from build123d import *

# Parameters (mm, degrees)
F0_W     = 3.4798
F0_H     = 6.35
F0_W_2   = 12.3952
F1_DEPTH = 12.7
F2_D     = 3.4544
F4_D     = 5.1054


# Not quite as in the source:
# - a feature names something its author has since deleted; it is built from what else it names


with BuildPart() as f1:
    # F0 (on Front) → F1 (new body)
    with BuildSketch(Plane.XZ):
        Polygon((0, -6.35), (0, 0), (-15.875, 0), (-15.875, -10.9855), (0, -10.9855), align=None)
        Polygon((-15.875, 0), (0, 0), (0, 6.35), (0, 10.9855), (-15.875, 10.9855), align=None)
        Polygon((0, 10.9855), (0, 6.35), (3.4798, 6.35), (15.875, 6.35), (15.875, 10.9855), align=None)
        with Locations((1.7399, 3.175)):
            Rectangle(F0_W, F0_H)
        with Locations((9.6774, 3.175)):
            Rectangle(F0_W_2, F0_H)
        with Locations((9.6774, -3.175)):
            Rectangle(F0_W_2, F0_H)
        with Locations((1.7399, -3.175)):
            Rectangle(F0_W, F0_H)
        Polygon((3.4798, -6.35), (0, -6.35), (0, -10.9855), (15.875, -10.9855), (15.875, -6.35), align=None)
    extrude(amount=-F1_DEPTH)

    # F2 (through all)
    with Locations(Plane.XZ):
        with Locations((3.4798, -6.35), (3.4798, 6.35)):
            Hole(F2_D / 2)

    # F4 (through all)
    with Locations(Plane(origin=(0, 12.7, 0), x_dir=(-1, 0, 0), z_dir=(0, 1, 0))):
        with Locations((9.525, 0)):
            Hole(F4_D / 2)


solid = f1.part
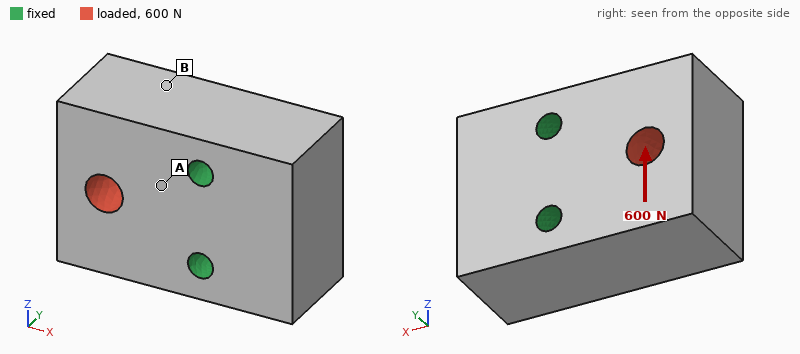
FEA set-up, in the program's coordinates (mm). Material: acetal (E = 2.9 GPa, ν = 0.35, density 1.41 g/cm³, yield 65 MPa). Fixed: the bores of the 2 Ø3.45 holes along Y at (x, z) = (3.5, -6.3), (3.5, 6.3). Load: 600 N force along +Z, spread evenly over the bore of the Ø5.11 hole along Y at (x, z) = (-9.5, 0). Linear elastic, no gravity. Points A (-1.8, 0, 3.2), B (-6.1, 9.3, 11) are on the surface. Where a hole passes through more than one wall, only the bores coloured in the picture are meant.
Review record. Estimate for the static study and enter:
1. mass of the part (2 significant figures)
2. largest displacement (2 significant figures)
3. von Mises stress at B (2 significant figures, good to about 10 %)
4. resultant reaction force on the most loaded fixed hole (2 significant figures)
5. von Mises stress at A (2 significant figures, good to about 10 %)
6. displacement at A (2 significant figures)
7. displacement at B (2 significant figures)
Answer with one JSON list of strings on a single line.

["12 g", "69 µm", "2.0 MPa", "590 N", "5.6 MPa", "13 µm", "39 µm"]
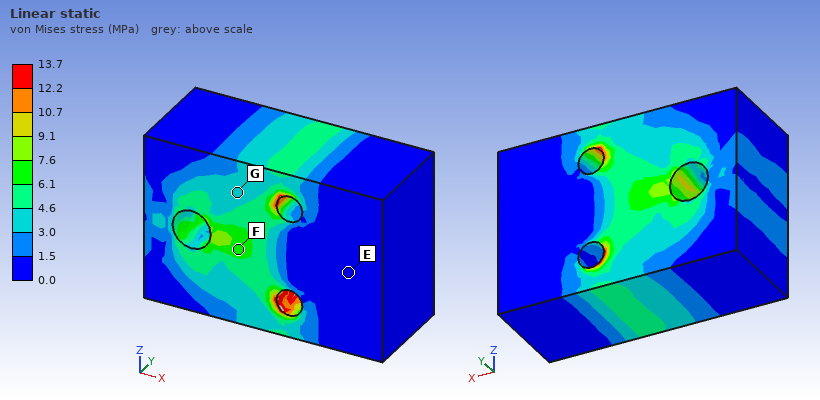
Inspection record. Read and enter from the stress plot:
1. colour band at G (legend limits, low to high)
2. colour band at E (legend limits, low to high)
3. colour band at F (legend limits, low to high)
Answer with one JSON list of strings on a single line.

["3.0 to 4.6 MPa", "0.0 to 1.5 MPa", "6.1 to 7.6 MPa"]
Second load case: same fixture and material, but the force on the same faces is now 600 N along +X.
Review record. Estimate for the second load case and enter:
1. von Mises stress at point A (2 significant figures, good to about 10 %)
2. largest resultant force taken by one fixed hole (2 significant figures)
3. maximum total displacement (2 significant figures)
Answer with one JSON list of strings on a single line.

["2.8 MPa", "310 N", "22 µm"]
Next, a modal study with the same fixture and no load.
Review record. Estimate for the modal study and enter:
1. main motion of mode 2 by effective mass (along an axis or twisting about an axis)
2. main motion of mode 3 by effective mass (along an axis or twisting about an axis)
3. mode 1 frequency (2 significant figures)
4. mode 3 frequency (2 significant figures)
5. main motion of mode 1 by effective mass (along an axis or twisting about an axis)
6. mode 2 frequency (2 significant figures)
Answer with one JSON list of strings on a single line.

["along Z", "twisting about X", "6200 Hz", "9600 Hz", "along Y", "7700 Hz"]
